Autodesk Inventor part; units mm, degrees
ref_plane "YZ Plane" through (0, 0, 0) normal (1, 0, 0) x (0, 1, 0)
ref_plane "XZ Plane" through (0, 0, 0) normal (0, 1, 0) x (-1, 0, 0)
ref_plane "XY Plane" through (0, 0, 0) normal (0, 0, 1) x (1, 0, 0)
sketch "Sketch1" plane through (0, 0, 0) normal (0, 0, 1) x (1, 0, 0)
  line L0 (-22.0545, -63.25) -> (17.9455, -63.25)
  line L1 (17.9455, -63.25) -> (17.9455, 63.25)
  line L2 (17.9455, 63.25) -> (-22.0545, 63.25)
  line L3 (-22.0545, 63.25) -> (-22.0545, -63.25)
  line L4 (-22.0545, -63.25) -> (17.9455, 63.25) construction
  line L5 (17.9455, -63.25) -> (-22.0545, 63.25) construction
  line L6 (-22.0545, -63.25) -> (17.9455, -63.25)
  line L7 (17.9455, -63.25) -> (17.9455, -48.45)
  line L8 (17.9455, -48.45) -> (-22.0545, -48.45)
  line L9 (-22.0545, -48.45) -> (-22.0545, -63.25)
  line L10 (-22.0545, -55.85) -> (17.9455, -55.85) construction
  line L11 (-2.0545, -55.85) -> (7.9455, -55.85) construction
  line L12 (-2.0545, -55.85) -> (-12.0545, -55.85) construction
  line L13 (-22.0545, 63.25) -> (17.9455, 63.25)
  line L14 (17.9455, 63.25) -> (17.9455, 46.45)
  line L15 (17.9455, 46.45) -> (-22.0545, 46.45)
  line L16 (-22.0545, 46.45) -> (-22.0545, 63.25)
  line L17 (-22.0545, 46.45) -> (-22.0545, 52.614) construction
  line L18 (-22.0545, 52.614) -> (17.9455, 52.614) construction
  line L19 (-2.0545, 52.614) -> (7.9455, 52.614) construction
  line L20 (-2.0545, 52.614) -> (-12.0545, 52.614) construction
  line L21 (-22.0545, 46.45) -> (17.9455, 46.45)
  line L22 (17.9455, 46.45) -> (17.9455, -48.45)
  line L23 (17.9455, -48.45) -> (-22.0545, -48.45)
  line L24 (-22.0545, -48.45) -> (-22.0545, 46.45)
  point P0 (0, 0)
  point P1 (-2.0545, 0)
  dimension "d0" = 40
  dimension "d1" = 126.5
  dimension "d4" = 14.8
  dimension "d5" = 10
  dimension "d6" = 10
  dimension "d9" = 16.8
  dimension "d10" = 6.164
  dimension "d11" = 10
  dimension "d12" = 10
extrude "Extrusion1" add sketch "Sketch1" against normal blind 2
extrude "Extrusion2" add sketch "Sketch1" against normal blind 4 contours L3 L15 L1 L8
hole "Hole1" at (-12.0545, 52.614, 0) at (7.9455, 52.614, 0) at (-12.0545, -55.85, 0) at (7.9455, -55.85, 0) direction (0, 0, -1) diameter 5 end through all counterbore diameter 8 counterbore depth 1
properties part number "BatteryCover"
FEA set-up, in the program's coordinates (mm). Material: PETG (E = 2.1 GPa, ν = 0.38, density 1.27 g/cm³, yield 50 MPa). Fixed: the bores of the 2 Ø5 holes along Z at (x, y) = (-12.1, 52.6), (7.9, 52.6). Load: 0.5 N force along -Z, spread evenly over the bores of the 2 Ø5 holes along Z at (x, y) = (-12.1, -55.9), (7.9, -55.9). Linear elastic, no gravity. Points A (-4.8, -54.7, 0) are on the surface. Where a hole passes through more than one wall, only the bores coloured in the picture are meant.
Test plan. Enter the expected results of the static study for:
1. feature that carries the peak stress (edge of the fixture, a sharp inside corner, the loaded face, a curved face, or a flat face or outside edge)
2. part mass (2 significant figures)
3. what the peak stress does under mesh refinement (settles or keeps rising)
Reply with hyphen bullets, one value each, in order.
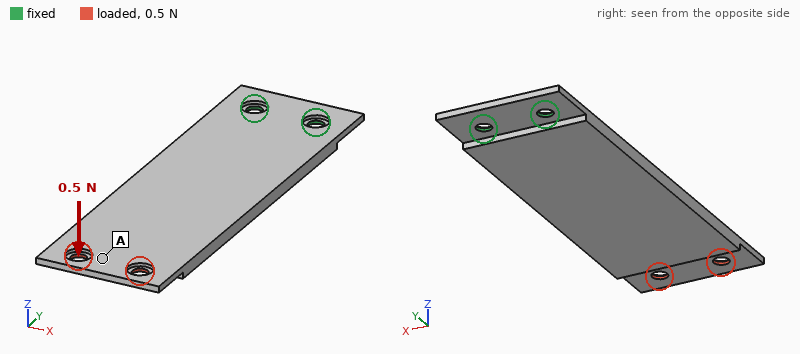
- edge of the fixture
- 22 g
- keeps rising
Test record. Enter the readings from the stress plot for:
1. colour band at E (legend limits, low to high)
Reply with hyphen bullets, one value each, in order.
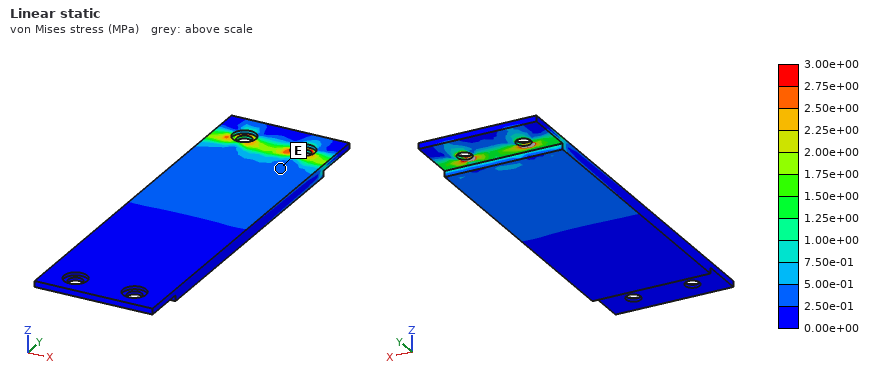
- 2.50e-01 to 5.00e-01 MPa
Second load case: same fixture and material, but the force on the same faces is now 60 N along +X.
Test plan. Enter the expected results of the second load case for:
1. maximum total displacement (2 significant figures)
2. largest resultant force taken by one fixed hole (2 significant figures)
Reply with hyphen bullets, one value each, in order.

- 1.3 mm
- 290 N
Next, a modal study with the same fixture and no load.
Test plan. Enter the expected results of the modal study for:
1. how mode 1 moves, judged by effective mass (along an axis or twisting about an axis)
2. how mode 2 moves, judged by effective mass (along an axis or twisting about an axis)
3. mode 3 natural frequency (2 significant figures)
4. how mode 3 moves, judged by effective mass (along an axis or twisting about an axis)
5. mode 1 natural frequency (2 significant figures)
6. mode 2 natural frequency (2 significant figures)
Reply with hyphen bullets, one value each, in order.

- along Z
- twisting about Y
- 340 Hz
- along Z
- 39 Hz
- 330 Hz
